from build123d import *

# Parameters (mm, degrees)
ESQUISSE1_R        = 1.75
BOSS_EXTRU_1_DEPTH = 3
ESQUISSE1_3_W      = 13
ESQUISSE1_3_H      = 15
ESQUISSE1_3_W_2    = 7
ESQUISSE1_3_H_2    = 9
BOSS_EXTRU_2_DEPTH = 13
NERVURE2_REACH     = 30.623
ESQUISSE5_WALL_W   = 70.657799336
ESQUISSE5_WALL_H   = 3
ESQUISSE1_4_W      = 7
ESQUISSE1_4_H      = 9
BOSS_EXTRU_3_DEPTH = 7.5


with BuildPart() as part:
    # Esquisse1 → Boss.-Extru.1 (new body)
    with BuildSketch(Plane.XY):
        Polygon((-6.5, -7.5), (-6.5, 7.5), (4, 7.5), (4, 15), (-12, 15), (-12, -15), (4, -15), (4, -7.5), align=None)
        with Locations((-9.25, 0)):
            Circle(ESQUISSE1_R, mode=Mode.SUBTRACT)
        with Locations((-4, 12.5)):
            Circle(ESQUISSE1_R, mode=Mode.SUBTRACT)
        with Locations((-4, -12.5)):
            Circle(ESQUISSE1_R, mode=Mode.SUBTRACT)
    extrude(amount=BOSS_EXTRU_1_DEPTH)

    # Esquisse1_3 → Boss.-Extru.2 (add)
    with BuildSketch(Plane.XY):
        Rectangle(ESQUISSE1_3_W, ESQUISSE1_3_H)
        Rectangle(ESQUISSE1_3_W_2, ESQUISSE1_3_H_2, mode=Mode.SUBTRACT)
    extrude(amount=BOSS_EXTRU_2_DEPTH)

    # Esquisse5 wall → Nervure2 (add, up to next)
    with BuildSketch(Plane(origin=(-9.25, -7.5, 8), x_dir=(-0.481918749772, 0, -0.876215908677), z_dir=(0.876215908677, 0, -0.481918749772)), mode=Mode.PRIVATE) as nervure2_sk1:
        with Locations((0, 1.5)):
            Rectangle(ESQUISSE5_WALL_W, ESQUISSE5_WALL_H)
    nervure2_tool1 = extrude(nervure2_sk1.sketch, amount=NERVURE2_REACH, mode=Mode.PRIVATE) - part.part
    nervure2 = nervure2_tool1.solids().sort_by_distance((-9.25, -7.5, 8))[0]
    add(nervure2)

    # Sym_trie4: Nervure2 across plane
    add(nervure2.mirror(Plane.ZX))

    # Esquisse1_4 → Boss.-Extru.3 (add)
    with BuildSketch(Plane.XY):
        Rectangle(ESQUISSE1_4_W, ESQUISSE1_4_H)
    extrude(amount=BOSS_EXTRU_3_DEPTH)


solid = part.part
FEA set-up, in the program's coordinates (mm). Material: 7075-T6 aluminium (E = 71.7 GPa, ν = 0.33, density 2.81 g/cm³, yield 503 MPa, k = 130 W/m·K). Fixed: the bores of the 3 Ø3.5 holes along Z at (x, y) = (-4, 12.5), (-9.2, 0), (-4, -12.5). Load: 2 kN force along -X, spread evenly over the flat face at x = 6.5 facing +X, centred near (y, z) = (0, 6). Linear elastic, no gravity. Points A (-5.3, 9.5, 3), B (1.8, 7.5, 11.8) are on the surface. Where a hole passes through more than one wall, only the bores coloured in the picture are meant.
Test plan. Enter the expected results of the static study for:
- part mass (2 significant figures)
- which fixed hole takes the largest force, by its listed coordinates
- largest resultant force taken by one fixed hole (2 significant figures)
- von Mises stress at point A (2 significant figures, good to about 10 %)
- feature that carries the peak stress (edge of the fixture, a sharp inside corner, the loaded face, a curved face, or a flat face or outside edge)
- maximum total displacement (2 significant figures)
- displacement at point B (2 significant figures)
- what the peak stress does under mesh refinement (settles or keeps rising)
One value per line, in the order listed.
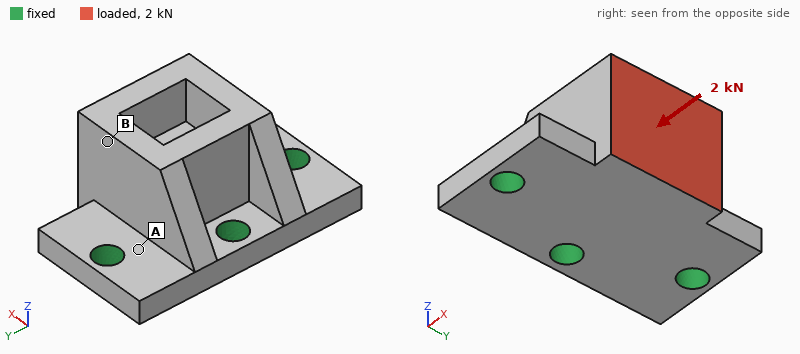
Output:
9.1 g
(-9.2, 0)
1.5 kN
69 MPa
edge of the fixture
60 µm
41 µm
keeps rising
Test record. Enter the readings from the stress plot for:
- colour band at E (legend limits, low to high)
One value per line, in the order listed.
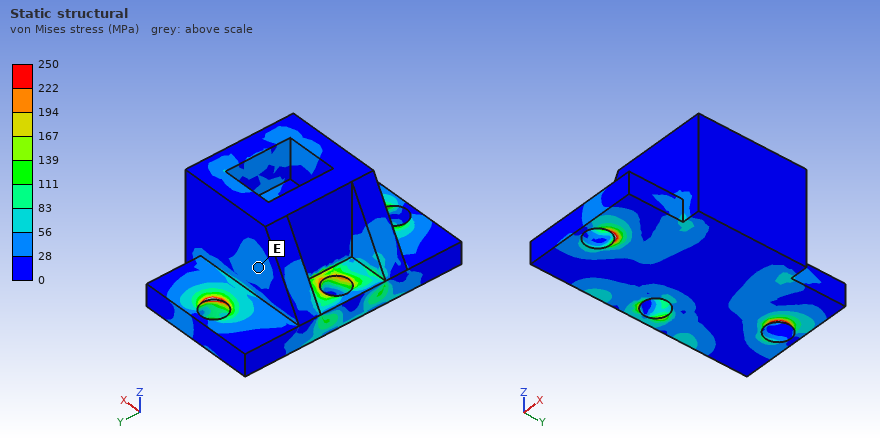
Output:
28 to 56 MPa
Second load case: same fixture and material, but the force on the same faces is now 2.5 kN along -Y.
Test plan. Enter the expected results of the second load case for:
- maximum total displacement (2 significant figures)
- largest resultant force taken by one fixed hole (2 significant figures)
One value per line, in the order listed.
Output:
34 µm
1.6 kN
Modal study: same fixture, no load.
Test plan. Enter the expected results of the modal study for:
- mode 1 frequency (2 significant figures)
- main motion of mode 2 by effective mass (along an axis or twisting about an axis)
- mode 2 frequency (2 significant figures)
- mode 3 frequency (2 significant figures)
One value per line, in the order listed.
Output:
12 kHz
along Y
26 kHz
40 kHz
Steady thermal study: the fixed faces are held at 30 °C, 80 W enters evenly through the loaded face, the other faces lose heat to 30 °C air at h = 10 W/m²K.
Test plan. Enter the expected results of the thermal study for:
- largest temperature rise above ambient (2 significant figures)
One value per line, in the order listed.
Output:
78 K
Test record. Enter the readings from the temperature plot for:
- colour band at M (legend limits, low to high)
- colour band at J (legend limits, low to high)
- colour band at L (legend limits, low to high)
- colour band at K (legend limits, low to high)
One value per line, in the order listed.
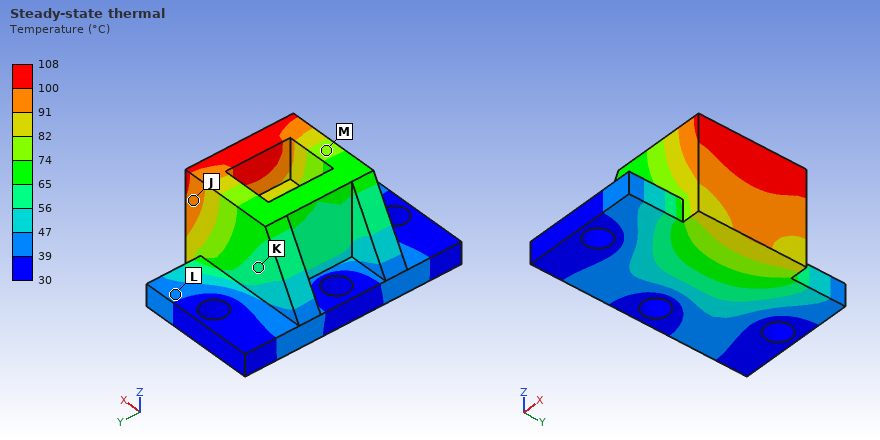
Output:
74 to 82 °C
91 to 100 °C
39 to 47 °C
56 to 65 °C
